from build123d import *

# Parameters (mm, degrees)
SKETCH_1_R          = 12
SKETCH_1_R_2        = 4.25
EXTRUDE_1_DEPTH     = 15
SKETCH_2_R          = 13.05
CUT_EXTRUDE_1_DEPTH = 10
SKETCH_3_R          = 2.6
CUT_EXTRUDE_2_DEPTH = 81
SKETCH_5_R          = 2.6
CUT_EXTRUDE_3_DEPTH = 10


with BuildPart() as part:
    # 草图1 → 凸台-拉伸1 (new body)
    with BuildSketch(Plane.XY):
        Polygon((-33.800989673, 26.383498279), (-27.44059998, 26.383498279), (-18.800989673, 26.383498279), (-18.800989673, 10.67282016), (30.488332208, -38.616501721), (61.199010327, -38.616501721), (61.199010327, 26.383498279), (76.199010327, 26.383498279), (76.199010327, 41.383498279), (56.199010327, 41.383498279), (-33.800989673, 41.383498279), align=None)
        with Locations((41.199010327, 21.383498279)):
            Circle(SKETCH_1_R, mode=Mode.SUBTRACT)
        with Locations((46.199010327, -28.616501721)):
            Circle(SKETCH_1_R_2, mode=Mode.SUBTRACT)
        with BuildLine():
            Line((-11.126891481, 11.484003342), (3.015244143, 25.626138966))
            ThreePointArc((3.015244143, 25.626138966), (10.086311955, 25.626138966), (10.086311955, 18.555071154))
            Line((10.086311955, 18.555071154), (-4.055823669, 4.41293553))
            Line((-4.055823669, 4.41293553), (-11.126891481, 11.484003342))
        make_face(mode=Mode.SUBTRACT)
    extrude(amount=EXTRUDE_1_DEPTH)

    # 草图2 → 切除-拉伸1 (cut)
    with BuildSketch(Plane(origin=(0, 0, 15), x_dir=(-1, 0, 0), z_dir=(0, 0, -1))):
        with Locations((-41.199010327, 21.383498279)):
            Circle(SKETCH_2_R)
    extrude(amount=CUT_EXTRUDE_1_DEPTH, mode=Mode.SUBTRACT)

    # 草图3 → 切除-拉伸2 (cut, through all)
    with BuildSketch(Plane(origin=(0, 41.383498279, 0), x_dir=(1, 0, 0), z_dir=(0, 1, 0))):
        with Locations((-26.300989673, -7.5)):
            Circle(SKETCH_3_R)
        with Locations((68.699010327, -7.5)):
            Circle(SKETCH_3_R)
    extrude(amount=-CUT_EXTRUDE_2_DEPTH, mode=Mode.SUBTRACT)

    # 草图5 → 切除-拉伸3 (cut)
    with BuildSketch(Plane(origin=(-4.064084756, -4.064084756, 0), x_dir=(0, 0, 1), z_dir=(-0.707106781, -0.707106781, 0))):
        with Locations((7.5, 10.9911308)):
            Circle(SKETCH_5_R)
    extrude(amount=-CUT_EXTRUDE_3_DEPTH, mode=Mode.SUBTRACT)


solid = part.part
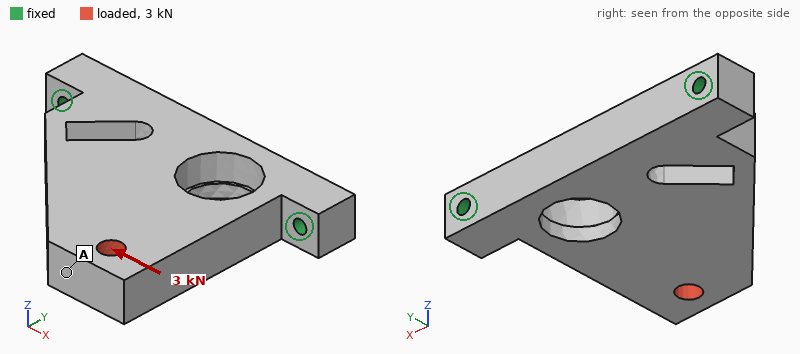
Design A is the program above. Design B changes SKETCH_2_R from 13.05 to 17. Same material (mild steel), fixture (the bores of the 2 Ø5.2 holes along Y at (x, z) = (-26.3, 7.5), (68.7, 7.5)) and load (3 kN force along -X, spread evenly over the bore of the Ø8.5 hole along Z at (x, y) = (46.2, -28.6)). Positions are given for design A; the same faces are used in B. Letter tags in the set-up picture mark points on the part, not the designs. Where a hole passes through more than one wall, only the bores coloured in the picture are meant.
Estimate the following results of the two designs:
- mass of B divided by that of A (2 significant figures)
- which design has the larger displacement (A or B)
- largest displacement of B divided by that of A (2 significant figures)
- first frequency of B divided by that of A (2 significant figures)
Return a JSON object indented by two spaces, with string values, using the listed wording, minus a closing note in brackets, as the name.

{
  "mass of B divided by that of A": "0.95",
  "which design has the larger displacement": "B",
  "largest displacement of B divided by that of A": "1.2",
  "first frequency of B divided by that of A": "0.94"
}
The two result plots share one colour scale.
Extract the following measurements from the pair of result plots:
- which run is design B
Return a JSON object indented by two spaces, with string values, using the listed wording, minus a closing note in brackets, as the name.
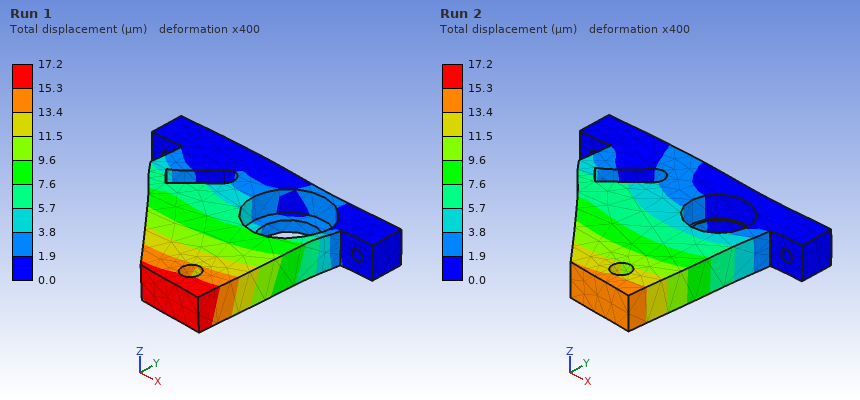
{
  "which run is design B": "Run 1"
}
